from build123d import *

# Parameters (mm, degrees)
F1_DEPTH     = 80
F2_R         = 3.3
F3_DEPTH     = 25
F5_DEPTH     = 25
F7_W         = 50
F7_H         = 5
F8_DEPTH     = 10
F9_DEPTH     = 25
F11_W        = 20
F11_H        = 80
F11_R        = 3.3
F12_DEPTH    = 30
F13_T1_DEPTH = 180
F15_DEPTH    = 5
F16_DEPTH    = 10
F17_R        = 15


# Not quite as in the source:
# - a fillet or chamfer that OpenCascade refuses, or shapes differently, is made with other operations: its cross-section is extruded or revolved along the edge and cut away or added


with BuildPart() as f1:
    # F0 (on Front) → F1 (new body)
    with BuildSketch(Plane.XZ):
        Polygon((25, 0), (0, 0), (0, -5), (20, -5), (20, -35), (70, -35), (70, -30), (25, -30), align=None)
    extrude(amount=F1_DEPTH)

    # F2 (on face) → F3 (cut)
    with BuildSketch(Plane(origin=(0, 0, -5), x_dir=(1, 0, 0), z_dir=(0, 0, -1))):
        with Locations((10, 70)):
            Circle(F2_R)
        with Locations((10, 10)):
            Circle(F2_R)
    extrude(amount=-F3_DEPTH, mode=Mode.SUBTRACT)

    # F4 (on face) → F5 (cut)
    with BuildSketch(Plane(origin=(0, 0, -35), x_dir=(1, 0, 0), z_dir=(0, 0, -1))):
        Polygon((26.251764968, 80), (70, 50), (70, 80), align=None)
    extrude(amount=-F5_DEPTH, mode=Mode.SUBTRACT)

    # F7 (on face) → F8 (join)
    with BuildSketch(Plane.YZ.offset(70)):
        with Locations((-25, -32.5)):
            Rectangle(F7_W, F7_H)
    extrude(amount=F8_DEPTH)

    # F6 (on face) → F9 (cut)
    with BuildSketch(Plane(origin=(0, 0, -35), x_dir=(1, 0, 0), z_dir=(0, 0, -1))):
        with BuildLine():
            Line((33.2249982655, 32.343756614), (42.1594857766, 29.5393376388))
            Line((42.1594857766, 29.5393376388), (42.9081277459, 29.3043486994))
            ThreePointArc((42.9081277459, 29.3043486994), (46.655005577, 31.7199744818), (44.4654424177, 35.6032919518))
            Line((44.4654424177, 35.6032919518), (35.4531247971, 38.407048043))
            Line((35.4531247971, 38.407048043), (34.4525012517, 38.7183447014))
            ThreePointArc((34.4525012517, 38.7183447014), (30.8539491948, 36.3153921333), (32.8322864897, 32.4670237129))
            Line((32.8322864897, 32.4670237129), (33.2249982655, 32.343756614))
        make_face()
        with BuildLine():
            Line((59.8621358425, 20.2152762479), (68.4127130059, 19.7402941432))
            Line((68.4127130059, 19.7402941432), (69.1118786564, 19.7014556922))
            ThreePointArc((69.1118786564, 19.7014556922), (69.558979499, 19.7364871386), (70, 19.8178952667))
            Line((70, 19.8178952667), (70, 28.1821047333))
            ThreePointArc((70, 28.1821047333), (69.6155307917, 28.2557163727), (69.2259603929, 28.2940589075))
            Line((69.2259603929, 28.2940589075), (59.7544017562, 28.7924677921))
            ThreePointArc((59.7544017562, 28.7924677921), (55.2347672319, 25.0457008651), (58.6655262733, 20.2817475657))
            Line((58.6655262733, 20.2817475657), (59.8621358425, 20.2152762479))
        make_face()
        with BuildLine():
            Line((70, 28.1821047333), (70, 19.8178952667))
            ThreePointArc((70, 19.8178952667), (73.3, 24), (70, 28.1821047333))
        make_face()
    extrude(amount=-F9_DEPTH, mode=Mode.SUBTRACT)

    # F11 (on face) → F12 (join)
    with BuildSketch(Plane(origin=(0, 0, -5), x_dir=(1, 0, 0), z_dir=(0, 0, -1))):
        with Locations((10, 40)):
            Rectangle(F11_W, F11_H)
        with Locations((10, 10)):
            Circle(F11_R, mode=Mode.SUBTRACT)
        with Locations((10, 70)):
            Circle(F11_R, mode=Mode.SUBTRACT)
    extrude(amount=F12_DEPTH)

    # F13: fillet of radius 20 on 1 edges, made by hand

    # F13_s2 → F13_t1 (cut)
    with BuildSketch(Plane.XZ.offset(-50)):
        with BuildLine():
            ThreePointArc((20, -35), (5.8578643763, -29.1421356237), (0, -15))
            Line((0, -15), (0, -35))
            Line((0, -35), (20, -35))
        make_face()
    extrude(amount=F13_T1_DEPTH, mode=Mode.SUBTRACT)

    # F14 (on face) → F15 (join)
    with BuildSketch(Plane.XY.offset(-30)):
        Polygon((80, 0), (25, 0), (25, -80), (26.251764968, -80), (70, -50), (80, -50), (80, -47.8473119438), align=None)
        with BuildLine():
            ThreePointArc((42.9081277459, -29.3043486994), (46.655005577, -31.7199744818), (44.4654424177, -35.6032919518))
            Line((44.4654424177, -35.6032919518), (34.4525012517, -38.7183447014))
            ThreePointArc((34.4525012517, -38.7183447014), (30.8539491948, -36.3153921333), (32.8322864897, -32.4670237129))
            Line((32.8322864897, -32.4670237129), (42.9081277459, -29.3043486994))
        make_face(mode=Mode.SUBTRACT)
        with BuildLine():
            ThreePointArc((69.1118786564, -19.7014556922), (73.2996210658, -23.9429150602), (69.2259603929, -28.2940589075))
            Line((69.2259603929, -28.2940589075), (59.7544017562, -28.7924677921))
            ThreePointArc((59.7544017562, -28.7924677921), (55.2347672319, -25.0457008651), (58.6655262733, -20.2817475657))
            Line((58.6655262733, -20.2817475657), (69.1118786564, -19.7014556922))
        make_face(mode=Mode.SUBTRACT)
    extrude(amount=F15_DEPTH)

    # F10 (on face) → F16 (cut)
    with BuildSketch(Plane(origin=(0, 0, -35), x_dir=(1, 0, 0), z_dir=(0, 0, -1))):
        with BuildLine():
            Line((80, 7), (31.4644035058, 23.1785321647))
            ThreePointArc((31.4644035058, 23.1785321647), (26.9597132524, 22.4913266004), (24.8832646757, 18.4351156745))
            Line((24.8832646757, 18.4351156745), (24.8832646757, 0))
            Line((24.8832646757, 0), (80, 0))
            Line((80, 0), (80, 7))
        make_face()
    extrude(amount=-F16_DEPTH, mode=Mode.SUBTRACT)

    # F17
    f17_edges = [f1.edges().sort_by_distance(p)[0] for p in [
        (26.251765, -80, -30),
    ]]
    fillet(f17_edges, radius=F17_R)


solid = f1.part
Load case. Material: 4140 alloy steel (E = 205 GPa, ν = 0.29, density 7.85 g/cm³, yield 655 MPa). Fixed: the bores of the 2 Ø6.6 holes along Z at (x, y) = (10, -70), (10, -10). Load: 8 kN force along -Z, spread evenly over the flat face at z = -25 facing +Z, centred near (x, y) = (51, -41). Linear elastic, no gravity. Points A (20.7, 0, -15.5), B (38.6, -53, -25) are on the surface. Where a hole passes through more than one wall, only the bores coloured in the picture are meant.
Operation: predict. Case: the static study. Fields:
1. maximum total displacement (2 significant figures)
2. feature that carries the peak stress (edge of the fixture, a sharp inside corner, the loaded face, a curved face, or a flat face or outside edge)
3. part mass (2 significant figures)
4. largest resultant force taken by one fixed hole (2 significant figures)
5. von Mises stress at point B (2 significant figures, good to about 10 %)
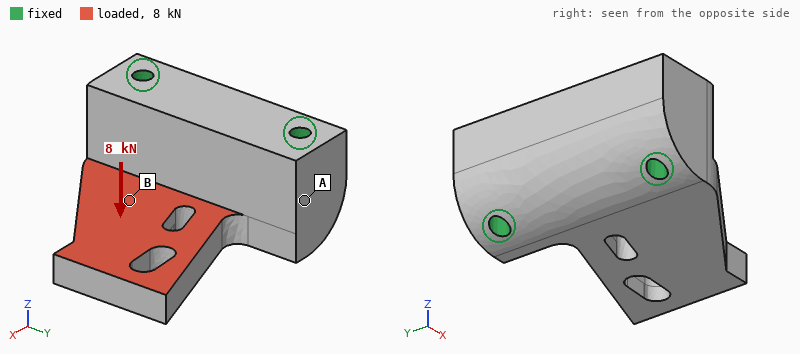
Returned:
0.38 mm
a curved face
660 g
4.2 kN
160 MPa
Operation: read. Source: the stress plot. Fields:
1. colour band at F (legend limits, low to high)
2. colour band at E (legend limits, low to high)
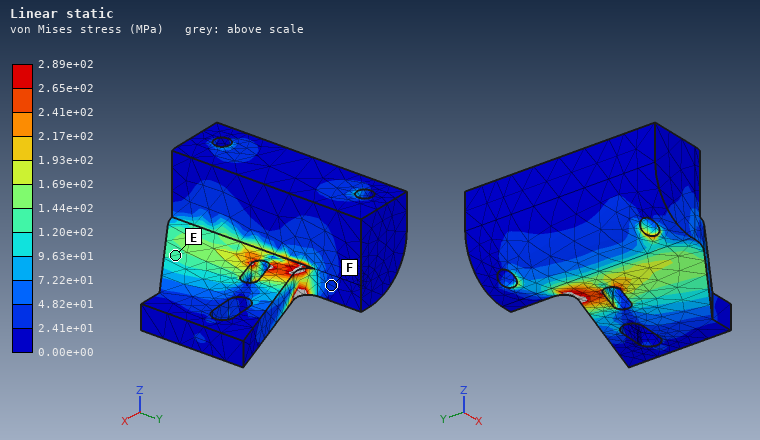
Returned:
2.41e+01 to 4.82e+01 MPa
1.20e+02 to 1.44e+02 MPa
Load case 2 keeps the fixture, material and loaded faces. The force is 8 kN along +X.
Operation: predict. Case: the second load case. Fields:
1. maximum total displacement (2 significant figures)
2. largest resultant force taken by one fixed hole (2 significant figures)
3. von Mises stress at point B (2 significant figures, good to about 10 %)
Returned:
63 µm
4.5 kN
44 MPa
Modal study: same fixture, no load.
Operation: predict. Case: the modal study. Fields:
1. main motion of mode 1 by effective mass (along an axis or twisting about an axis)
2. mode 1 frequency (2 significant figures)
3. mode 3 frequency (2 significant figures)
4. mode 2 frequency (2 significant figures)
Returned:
along Z
2300 Hz
6900 Hz
6300 Hz
